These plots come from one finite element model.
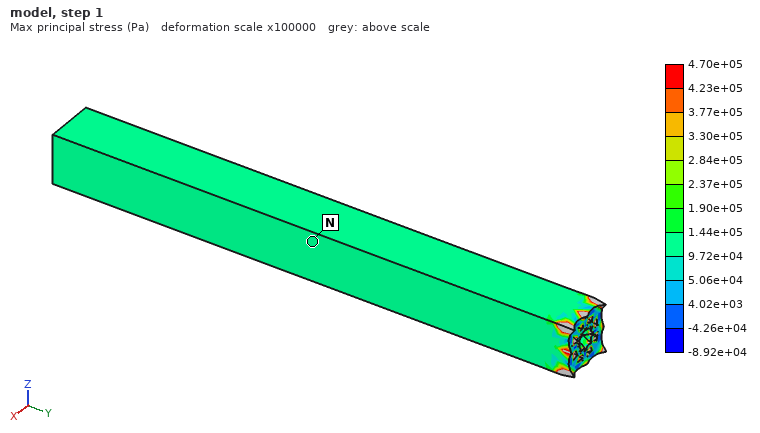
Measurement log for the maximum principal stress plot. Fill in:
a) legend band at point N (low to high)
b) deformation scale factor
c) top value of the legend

9.72e+04 to 1.44e+05 Pa
100000
4.70e+05 Pa
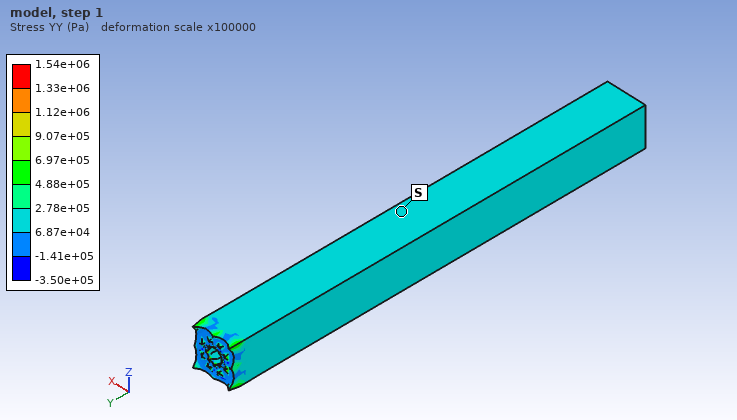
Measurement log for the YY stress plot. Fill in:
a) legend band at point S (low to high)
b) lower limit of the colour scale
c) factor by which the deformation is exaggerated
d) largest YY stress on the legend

6.87e+04 to 2.78e+05 Pa
-3.50e+05 Pa
100000
1.54e+06 Pa
